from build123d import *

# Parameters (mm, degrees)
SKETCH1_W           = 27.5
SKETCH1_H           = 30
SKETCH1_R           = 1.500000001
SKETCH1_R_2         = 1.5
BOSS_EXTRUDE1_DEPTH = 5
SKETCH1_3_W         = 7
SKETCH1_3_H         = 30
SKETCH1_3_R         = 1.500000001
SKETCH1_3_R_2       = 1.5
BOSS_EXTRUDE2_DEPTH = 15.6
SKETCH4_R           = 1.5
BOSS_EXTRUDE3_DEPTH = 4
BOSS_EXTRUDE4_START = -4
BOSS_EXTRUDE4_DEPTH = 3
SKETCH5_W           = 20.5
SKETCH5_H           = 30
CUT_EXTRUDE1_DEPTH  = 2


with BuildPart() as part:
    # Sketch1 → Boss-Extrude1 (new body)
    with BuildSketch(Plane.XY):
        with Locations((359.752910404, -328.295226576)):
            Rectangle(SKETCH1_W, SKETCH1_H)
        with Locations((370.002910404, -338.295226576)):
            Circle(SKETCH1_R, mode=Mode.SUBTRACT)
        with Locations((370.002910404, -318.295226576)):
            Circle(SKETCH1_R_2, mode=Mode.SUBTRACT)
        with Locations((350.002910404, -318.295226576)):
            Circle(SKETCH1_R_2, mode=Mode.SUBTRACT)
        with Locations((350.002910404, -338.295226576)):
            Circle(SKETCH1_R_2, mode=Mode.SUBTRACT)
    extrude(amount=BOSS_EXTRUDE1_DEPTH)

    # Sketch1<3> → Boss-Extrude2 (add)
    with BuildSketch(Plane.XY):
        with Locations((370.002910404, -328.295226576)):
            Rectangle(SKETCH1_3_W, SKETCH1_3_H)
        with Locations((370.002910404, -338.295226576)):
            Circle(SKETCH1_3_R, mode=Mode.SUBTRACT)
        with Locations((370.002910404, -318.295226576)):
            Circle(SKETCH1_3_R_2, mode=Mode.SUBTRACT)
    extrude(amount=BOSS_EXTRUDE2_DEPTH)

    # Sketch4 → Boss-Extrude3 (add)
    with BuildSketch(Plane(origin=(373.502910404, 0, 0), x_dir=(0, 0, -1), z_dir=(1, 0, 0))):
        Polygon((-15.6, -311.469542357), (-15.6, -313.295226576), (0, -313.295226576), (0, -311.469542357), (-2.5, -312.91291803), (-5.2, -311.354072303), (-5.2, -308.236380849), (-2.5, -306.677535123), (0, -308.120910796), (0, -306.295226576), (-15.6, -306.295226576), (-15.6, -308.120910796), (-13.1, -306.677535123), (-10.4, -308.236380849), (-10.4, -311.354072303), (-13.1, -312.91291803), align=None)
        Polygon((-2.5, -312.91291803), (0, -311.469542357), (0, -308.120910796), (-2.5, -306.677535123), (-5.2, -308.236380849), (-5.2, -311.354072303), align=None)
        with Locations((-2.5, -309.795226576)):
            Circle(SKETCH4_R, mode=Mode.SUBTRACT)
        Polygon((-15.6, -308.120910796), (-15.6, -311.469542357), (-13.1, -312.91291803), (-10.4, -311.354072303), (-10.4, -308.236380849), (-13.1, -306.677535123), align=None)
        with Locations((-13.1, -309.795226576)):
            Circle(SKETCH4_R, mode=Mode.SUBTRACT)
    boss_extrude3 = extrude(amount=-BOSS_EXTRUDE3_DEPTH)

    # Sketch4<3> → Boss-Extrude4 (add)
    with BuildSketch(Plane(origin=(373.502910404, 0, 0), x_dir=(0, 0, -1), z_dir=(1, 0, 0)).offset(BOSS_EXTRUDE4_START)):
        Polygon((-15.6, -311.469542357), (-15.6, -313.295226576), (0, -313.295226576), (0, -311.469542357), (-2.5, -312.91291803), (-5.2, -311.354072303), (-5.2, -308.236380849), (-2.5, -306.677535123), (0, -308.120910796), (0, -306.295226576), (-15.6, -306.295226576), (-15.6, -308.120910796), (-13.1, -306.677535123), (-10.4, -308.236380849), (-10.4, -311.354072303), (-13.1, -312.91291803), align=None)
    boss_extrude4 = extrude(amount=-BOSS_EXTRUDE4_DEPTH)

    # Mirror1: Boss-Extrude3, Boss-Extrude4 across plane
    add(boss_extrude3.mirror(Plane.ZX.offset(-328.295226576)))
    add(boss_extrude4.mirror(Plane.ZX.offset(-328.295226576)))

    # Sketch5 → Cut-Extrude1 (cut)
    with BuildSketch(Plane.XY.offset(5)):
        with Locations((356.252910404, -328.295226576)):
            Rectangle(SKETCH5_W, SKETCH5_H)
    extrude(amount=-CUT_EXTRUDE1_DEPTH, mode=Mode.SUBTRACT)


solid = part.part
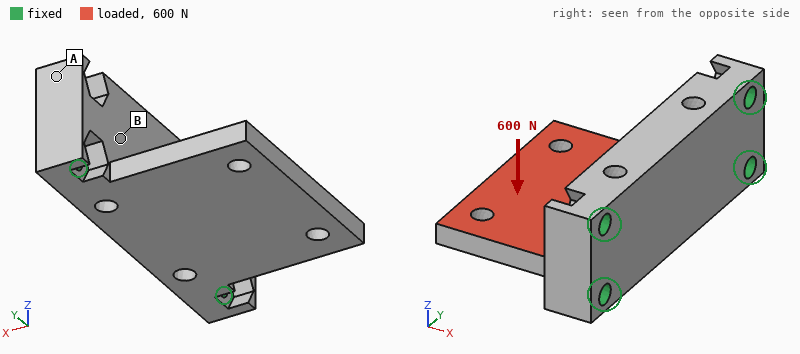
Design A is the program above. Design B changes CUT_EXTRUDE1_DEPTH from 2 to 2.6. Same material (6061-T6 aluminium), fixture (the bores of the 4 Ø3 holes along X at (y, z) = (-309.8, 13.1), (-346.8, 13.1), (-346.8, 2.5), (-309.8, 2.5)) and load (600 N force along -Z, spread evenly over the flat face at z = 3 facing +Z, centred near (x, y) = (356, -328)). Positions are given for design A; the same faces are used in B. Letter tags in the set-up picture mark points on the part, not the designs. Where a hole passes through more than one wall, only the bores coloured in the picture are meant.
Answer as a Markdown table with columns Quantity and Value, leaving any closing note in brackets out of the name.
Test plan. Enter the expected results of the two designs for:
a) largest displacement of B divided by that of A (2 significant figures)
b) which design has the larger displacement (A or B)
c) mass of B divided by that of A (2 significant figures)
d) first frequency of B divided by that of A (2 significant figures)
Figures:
| Quantity | Value |
|---|---|
| largest displacement of B divided by that of A | 1.7 |
| which design has the larger displacement | B |
| mass of B divided by that of A | 0.94 |
| first frequency of B divided by that of A | 0.86 |
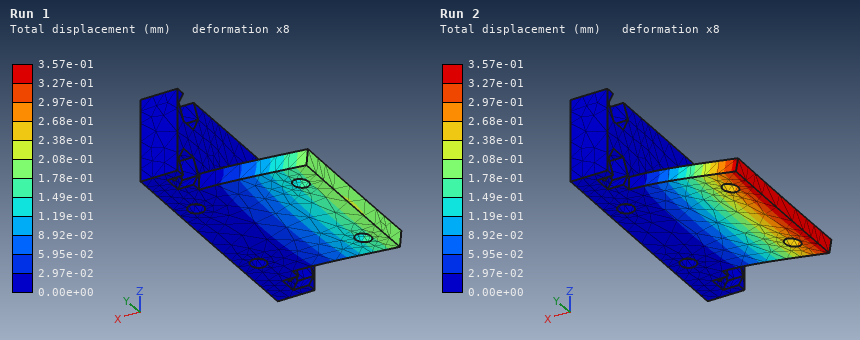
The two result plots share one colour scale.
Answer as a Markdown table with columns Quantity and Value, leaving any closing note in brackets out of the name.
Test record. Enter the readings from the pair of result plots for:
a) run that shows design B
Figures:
| Quantity | Value |
|---|---|
| run that shows design B | Run 2 |
